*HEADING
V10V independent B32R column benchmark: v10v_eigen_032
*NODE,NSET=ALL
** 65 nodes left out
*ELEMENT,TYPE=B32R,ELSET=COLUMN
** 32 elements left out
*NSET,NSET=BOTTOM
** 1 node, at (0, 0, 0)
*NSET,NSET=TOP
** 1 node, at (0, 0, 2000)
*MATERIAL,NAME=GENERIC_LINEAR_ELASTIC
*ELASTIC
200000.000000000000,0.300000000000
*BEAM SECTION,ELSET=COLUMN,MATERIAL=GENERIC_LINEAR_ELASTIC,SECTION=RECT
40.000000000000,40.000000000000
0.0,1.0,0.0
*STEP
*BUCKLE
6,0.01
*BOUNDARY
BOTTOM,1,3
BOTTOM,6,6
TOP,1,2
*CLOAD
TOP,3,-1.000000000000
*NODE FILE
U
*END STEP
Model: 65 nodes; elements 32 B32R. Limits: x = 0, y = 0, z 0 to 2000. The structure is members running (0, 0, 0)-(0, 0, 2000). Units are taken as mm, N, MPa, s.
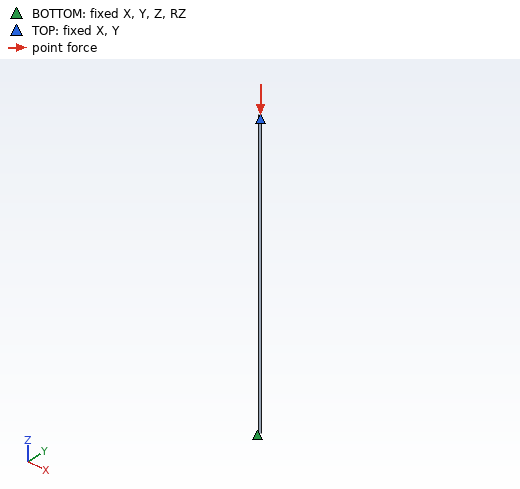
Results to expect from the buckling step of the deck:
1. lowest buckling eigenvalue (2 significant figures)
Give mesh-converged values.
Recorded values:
1.1e+05
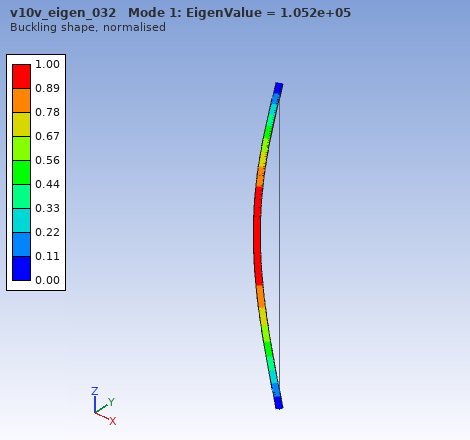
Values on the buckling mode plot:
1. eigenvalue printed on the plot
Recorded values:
1.052e+05
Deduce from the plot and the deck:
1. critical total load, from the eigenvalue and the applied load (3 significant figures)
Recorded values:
1.05e+05 N
